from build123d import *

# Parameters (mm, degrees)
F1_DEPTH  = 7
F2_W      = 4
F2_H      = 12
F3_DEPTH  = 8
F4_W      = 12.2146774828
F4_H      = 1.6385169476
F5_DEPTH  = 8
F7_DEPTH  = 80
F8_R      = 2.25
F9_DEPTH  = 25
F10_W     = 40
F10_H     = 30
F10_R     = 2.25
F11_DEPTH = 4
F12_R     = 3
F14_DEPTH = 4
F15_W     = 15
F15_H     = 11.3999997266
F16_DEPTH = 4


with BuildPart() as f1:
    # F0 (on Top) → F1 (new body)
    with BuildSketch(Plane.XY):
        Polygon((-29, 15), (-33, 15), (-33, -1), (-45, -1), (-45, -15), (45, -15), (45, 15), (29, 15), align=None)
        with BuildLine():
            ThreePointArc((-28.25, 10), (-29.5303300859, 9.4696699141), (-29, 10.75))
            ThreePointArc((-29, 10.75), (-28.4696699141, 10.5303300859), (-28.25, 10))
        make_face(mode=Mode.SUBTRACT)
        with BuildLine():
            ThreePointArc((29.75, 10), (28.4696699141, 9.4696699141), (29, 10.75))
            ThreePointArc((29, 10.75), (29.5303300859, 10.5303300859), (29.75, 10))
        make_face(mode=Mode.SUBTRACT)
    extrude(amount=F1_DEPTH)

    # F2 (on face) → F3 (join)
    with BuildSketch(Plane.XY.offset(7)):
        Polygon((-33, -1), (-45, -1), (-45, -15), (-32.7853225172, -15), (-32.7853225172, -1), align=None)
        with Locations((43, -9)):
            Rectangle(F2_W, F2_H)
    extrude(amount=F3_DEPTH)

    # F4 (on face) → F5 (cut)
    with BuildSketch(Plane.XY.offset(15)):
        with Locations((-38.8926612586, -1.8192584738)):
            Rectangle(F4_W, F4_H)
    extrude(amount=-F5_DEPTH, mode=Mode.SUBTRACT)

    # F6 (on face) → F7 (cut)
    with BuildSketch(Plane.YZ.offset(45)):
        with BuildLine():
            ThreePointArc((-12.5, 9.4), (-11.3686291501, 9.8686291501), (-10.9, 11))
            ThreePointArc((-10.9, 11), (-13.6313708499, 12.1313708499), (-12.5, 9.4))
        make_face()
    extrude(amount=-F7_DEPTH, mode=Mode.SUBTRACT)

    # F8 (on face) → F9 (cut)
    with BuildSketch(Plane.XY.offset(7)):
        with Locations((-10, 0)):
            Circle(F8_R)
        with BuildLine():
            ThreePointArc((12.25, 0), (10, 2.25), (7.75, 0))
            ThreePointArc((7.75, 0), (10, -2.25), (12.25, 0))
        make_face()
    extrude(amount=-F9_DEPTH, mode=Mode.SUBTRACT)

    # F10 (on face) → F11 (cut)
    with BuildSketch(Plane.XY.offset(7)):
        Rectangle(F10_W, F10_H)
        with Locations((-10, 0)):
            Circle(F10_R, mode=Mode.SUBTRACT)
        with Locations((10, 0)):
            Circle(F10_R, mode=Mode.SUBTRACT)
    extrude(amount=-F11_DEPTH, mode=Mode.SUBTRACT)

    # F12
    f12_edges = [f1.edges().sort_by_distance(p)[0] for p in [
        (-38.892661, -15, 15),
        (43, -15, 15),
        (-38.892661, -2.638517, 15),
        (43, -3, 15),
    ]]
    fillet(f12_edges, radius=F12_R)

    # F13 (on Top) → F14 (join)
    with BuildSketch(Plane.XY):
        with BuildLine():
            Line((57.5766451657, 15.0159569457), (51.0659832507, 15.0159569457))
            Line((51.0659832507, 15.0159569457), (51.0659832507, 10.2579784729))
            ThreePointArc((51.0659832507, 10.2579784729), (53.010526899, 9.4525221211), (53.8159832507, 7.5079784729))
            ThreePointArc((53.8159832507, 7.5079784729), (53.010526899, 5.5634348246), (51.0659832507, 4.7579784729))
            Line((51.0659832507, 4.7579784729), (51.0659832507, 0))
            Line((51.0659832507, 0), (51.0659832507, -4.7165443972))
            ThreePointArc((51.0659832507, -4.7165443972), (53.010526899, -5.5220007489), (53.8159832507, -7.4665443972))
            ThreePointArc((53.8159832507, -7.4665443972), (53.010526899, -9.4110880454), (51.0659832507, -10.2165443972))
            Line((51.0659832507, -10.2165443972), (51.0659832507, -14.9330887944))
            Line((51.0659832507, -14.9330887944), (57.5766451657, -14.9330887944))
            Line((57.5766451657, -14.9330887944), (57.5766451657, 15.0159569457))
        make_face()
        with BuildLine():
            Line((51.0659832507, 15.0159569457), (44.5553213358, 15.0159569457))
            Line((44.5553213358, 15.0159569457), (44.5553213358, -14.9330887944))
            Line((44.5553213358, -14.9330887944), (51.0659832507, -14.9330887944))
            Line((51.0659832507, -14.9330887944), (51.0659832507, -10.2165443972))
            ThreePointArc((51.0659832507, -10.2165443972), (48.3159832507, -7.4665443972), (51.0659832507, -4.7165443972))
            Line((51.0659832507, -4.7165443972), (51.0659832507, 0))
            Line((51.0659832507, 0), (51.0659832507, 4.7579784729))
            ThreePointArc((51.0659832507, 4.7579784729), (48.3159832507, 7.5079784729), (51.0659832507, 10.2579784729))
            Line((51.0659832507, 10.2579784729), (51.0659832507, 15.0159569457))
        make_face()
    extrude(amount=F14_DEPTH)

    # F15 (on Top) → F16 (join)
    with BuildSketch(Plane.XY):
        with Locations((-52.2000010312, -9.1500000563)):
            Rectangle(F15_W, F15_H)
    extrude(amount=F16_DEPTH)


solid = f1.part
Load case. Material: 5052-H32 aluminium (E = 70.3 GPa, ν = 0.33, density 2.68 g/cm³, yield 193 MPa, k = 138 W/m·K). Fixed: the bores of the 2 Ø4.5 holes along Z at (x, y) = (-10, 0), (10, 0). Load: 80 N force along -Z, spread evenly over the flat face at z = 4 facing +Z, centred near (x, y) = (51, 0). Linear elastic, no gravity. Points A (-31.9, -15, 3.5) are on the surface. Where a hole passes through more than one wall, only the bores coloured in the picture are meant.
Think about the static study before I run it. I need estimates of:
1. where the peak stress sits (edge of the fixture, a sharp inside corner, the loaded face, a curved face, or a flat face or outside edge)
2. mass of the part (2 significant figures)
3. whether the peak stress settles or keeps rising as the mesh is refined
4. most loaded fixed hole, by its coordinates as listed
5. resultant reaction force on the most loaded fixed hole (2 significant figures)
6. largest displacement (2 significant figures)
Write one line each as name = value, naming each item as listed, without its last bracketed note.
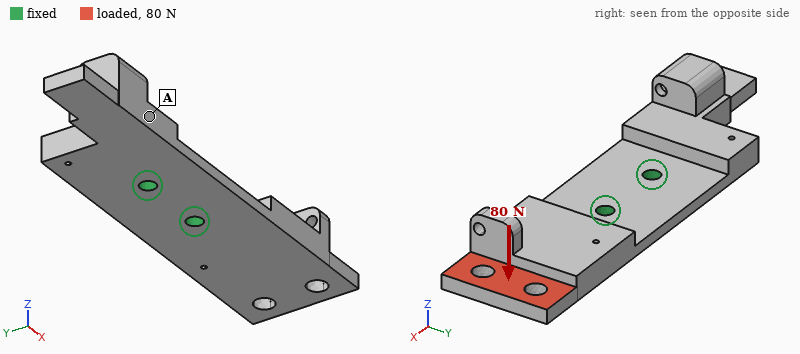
where the peak stress sits = edge of the fixture
mass of the part = 43 g
whether the peak stress settles or keeps rising as the mesh is refined = keeps rising
most loaded fixed hole, by its coordinates as listed = (10, 0)
resultant reaction force on the most loaded fixed hole = 130 N
largest displacement = 0.30 mm
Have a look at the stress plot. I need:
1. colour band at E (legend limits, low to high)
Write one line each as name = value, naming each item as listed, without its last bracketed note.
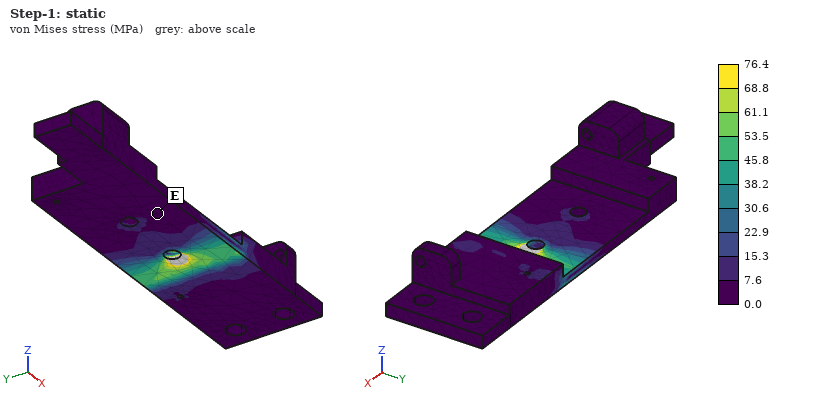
colour band at E = 0.0 to 7.6 MPa
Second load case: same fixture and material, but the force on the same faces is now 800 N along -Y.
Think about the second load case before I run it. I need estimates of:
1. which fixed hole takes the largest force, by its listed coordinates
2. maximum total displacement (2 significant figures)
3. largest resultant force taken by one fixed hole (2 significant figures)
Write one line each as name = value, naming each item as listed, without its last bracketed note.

which fixed hole takes the largest force, by its listed coordinates = (10, 0)
maximum total displacement = 0.12 mm
largest resultant force taken by one fixed hole = 2.1 kN
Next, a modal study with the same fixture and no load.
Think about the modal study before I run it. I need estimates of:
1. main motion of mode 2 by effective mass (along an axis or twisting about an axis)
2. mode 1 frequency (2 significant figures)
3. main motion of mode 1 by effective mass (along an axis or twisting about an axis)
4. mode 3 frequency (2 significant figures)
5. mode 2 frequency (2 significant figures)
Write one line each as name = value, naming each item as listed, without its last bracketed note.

main motion of mode 2 by effective mass = along Z
mode 1 frequency = 1000 Hz
main motion of mode 1 by effective mass = along Z
mode 3 frequency = 3500 Hz
mode 2 frequency = 1200 Hz
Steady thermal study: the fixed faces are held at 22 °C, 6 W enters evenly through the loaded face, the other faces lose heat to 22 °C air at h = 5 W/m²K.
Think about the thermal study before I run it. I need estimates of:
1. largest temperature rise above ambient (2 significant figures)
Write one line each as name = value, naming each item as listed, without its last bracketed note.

largest temperature rise above ambient = 15 K
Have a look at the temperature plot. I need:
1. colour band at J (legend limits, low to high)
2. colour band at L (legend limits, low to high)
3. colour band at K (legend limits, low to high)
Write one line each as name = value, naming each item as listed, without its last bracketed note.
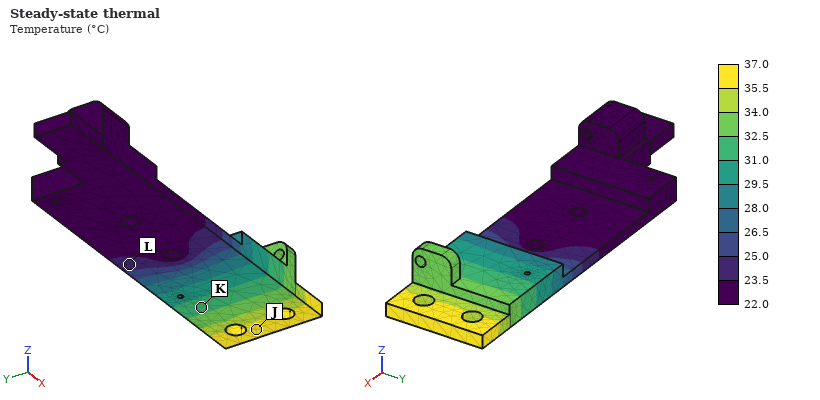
colour band at J = 35.5 to 37.0 °C
colour band at L = 23.5 to 25.0 °C
colour band at K = 31.0 to 32.5 °C
